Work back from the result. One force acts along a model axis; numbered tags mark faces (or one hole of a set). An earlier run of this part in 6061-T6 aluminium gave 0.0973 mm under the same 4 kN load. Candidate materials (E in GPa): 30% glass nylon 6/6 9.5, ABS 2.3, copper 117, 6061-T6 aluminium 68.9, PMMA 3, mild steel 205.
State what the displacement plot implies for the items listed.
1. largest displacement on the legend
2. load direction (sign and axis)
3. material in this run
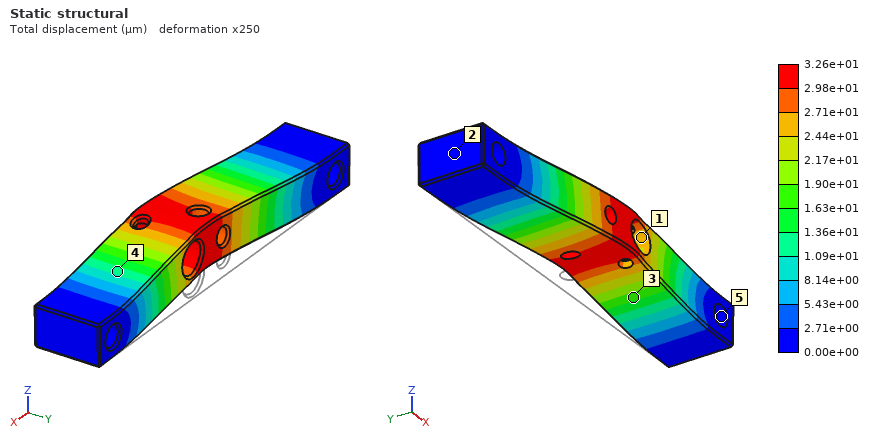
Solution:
3.26e+01 µm
+Z
mild steel
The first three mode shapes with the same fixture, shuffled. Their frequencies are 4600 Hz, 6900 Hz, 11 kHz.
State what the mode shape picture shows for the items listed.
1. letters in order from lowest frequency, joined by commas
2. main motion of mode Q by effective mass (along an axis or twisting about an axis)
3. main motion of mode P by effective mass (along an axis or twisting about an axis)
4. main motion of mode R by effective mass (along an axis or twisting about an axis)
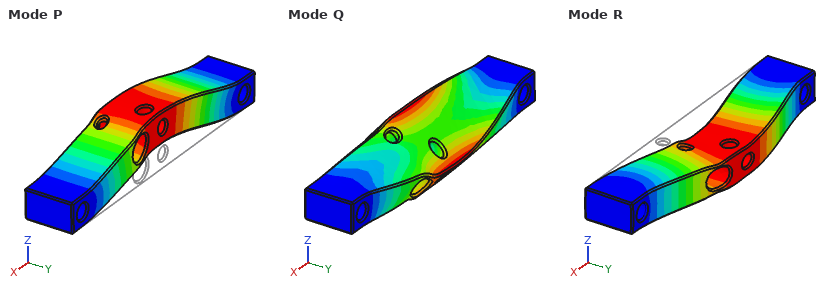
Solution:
P, R, Q
twisting about X
along Z
along Y
